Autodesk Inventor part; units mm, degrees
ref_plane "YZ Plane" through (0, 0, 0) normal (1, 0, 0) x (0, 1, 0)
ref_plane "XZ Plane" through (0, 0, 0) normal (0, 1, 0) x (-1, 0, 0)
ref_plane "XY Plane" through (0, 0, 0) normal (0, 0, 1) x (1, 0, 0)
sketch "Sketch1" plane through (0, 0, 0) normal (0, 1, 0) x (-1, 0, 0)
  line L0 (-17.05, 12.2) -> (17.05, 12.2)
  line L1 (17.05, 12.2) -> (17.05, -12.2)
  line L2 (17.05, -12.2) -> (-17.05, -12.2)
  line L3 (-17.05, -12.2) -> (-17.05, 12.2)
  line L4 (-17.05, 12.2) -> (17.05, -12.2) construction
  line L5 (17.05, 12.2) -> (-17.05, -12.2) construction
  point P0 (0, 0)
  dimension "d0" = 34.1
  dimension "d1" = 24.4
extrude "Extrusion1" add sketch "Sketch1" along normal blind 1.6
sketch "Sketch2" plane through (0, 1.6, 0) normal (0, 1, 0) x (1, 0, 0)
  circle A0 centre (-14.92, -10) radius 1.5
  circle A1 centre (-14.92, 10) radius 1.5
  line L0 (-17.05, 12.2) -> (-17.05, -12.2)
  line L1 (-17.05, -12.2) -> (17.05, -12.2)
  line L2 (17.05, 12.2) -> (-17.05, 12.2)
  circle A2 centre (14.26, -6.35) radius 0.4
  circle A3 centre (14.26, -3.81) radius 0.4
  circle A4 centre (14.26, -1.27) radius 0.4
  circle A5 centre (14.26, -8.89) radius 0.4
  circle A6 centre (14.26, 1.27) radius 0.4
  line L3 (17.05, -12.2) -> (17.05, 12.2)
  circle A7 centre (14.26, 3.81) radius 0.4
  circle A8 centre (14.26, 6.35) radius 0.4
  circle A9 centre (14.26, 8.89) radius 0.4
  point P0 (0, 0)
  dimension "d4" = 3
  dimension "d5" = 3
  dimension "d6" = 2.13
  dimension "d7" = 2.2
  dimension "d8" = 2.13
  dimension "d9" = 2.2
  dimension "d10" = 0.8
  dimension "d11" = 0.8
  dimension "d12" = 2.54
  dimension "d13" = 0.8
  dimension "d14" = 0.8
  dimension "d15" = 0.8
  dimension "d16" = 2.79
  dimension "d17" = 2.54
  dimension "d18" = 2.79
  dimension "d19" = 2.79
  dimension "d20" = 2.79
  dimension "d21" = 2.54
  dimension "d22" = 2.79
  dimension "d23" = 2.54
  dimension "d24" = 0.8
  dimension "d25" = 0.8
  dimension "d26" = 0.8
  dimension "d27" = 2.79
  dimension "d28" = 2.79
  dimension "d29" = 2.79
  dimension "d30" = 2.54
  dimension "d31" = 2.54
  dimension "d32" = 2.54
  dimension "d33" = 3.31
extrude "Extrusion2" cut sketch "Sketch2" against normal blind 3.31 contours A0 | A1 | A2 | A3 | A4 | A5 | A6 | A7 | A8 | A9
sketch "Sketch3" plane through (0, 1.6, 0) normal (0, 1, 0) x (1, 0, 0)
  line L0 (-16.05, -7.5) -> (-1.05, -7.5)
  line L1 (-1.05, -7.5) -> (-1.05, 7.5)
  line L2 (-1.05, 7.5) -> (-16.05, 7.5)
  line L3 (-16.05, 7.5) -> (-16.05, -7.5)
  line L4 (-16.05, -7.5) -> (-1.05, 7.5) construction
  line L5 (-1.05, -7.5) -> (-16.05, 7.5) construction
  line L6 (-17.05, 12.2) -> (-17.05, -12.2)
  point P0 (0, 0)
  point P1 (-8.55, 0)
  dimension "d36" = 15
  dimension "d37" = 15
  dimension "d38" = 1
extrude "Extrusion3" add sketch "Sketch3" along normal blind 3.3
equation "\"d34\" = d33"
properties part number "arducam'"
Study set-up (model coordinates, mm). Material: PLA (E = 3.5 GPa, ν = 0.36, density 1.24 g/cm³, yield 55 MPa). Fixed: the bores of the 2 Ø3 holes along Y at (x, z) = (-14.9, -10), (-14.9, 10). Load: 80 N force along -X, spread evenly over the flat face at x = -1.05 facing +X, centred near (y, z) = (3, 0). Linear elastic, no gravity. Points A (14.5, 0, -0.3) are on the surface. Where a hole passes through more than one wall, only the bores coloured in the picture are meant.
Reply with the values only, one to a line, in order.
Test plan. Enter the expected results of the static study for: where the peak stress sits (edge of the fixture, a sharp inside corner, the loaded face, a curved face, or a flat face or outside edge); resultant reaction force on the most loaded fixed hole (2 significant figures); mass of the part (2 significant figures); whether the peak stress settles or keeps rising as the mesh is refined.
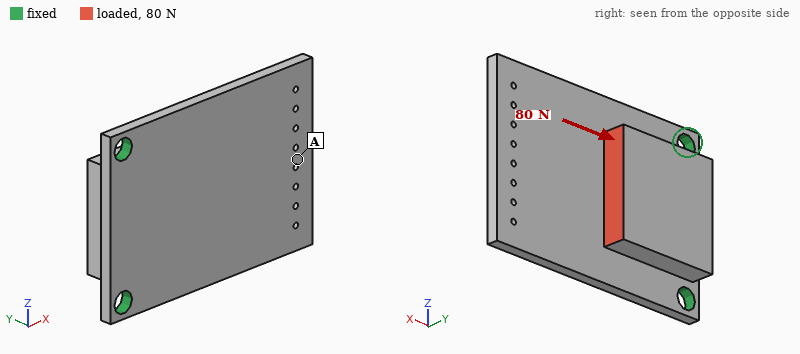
edge of the fixture
42 N
2.5 g
keeps rising
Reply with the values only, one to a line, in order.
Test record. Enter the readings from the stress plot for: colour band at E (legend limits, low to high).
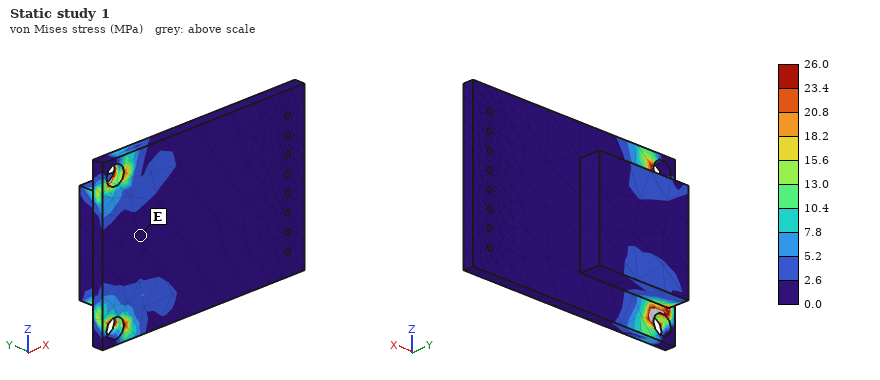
0.0 to 2.6 MPa
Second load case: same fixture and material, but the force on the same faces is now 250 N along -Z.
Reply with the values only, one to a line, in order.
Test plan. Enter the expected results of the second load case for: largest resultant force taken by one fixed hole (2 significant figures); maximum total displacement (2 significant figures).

210 N
0.12 mm
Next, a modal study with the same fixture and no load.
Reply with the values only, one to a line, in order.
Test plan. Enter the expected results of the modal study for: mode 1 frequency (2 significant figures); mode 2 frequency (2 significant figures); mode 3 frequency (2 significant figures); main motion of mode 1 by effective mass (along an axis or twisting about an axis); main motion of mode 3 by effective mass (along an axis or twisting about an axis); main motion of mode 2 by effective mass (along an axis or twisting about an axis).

700 Hz
2100 Hz
2600 Hz
along Y
along Y
twisting about X
